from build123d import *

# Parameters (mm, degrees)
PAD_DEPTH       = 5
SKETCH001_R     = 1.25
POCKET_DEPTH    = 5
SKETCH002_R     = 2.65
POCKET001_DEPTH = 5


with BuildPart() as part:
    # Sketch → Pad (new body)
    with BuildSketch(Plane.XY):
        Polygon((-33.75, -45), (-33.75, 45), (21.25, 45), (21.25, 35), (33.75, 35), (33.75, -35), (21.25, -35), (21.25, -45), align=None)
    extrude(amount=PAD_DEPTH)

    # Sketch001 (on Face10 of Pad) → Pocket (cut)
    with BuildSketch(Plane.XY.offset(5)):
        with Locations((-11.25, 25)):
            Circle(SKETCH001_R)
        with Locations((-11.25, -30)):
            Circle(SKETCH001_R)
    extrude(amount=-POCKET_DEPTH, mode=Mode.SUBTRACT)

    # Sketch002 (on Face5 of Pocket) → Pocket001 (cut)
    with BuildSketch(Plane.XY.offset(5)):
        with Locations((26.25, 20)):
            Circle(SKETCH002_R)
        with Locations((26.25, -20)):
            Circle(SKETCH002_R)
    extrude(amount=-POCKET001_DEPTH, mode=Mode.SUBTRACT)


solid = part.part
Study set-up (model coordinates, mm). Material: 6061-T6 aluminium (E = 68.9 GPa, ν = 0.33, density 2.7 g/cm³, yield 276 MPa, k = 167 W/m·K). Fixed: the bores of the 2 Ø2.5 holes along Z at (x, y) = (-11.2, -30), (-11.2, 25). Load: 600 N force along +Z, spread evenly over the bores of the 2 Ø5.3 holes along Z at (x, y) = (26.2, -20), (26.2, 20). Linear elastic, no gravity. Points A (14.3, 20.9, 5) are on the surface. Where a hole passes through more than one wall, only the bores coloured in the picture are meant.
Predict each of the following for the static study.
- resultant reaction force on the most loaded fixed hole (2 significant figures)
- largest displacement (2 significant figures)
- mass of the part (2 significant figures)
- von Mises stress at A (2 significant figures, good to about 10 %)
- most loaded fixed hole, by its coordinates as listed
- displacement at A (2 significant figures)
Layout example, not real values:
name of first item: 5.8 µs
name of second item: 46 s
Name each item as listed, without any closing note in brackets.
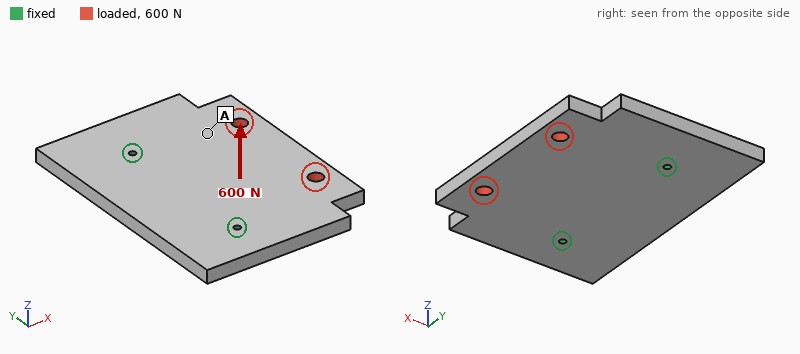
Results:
resultant reaction force on the most loaded fixed hole: 320 N
largest displacement: 0.37 mm
mass of the part: 78 g
von Mises stress at A: 21 MPa
most loaded fixed hole, by its coordinates as listed: (-11.2, 25)
displacement at A: 0.17 mm
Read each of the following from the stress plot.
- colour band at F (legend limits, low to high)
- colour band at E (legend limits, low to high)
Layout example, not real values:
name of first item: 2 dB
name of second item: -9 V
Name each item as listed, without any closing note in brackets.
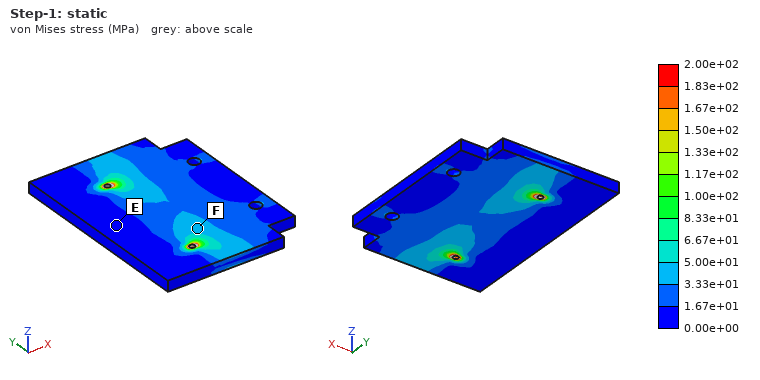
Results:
colour band at F: 3.33e+01 to 5.00e+01 MPa
colour band at E: 0.00e+00 to 1.67e+01 MPa
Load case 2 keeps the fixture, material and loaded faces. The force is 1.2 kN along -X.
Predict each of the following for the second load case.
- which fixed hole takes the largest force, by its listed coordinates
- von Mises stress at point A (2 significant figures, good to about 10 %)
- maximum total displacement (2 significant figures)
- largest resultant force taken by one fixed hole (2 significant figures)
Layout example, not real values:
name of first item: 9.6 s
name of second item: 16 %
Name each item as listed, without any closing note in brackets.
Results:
which fixed hole takes the largest force, by its listed coordinates: (-11.2, 25)
von Mises stress at point A: 5.4 MPa
maximum total displacement: 4.2 µm
largest resultant force taken by one fixed hole: 660 N
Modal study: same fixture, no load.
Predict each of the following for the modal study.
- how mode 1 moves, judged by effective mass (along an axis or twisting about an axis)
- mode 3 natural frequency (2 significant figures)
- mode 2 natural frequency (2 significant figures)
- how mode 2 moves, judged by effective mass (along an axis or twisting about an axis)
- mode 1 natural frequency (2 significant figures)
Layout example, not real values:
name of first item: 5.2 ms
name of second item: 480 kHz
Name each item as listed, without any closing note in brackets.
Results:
how mode 1 moves, judged by effective mass: along Z
mode 3 natural frequency: 4600 Hz
mode 2 natural frequency: 3200 Hz
how mode 2 moves, judged by effective mass: twisting about X
mode 1 natural frequency: 1600 Hz
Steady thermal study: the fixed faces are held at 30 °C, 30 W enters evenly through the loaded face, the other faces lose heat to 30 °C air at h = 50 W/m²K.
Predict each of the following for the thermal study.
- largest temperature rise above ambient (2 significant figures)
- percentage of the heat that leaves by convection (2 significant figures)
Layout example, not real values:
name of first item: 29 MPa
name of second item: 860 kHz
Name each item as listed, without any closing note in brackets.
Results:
largest temperature rise above ambient: 23 K
percentage of the heat that leaves by convection: 20 %
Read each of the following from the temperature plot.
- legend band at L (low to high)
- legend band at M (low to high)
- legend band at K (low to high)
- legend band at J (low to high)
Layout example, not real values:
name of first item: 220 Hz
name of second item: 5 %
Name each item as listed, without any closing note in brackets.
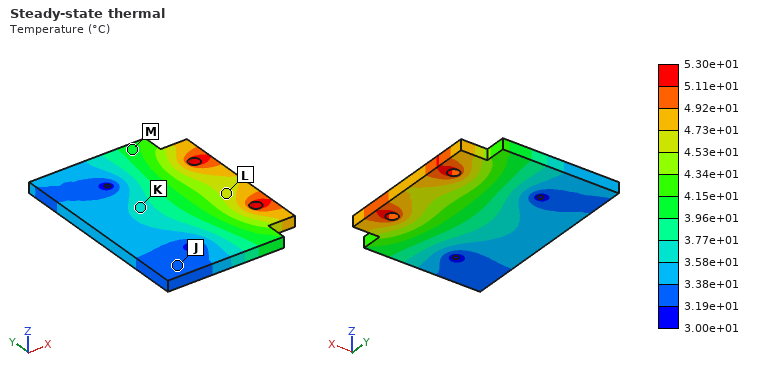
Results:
legend band at L: 4.53e+01 to 4.73e+01 °C
legend band at M: 3.96e+01 to 4.15e+01 °C
legend band at K: 3.58e+01 to 3.77e+01 °C
legend band at J: 3.19e+01 to 3.38e+01 °C
